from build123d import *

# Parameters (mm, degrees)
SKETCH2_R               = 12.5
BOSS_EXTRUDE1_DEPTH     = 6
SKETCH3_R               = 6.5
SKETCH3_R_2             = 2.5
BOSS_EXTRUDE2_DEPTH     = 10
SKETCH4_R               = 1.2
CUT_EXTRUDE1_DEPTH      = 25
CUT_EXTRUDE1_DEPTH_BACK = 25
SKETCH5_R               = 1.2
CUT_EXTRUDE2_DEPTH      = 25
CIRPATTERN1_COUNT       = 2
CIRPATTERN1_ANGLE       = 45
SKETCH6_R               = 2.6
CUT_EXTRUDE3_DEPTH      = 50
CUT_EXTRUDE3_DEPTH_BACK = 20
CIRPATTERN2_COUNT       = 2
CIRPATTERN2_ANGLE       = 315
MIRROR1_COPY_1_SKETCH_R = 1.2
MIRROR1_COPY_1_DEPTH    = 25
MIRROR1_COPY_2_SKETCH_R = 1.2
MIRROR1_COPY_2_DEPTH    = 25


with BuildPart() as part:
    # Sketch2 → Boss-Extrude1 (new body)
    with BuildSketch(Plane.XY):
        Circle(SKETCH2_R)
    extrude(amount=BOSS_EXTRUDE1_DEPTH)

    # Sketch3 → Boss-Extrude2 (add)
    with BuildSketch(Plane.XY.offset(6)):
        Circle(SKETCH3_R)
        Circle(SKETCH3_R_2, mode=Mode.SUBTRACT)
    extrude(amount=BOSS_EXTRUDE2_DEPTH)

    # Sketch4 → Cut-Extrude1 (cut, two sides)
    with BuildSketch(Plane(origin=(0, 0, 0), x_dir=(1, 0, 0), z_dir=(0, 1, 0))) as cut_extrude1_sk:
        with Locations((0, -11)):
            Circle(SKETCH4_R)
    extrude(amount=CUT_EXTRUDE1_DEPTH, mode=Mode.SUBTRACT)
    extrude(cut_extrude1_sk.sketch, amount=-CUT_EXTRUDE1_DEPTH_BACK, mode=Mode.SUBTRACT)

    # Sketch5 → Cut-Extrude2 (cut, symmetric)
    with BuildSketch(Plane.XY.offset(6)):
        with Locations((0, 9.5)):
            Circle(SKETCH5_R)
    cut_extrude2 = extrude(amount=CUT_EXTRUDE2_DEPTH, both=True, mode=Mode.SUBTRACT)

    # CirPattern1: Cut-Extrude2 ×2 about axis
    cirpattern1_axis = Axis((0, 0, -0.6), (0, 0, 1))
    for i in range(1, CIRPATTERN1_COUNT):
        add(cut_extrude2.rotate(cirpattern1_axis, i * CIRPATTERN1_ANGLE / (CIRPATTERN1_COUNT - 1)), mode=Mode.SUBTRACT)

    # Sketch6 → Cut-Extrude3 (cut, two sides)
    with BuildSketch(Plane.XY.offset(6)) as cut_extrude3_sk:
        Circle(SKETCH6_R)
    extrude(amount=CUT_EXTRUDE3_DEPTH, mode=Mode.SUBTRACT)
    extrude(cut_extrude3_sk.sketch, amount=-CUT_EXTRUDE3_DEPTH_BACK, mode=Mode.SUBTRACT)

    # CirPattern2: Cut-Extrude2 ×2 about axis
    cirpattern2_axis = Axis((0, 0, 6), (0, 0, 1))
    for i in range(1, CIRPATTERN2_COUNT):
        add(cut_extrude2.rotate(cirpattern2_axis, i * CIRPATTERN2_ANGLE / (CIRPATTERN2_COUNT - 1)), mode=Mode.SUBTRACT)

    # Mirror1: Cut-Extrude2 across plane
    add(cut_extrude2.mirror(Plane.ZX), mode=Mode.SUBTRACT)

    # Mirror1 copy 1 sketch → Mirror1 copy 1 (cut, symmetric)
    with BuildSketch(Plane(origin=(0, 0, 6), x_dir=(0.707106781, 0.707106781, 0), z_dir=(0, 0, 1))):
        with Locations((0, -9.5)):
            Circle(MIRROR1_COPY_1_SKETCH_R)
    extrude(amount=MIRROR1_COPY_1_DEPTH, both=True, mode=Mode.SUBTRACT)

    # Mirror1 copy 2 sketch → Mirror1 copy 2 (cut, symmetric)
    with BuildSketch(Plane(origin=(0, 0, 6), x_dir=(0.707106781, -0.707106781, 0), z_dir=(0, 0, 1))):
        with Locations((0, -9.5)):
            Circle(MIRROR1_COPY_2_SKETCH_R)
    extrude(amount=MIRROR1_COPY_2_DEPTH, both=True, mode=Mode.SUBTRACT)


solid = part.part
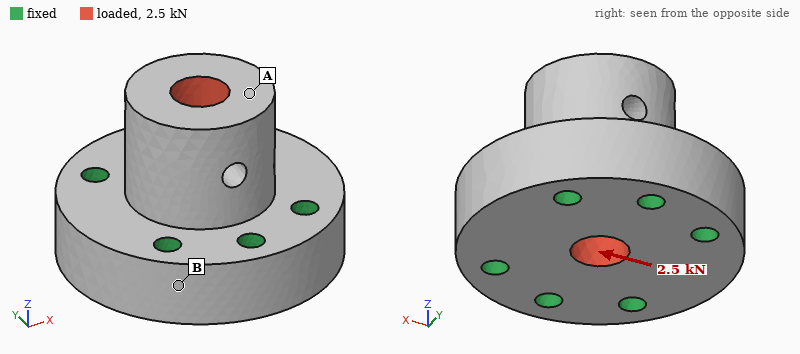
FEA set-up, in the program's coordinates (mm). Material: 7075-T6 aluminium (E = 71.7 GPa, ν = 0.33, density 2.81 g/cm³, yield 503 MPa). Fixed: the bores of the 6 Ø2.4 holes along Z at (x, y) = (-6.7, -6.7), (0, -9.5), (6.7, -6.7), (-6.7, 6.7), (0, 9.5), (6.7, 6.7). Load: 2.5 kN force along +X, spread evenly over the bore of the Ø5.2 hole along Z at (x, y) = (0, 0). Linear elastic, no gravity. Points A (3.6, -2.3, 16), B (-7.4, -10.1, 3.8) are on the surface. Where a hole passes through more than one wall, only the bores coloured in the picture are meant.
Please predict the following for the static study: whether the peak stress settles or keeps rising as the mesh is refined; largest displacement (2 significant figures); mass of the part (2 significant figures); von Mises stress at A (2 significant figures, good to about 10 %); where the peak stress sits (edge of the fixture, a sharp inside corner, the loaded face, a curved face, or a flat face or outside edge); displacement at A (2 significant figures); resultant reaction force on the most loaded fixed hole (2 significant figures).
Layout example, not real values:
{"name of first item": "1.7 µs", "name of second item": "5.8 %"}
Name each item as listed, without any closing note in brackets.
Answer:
{"whether the peak stress settles or keeps rising as the mesh is refined": "keeps rising", "largest displacement": "13 µm", "mass of the part": "10 g", "von Mises stress at A": "14 MPa", "where the peak stress sits": "edge of the fixture", "displacement at A": "12 µm", "resultant reaction force on the most loaded fixed hole": "720 N"}
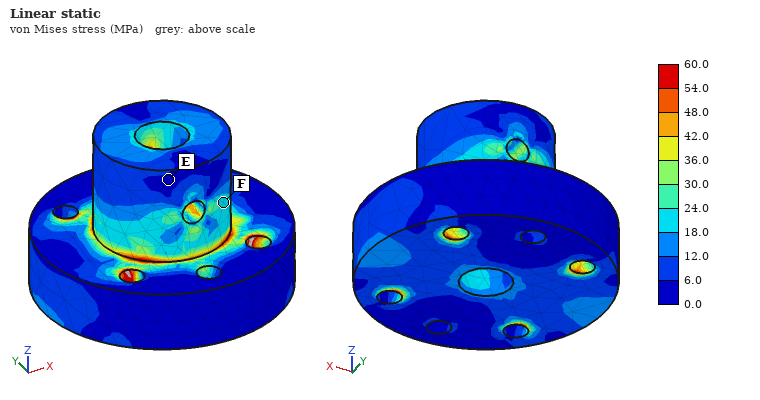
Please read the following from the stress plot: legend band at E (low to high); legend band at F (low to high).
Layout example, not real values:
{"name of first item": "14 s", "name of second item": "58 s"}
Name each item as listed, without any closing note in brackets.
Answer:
{"legend band at E": "0.0 to 6.0 MPa", "legend band at F": "18.0 to 24.0 MPa"}
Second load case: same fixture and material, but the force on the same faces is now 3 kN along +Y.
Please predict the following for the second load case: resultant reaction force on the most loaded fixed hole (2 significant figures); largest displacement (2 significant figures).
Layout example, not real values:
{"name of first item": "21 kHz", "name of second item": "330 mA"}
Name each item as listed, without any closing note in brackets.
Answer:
{"resultant reaction force on the most loaded fixed hole": "770 N", "largest displacement": "13 µm"}
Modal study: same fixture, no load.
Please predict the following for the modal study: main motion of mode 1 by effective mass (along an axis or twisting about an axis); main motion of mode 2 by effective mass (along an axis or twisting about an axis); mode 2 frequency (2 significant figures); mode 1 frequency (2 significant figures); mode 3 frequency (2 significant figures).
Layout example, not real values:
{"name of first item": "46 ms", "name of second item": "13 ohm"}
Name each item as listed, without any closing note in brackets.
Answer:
{"main motion of mode 1 by effective mass": "along X", "main motion of mode 2 by effective mass": "along Y", "mode 2 frequency": "42 kHz", "mode 1 frequency": "37 kHz", "mode 3 frequency": "65 kHz"}
